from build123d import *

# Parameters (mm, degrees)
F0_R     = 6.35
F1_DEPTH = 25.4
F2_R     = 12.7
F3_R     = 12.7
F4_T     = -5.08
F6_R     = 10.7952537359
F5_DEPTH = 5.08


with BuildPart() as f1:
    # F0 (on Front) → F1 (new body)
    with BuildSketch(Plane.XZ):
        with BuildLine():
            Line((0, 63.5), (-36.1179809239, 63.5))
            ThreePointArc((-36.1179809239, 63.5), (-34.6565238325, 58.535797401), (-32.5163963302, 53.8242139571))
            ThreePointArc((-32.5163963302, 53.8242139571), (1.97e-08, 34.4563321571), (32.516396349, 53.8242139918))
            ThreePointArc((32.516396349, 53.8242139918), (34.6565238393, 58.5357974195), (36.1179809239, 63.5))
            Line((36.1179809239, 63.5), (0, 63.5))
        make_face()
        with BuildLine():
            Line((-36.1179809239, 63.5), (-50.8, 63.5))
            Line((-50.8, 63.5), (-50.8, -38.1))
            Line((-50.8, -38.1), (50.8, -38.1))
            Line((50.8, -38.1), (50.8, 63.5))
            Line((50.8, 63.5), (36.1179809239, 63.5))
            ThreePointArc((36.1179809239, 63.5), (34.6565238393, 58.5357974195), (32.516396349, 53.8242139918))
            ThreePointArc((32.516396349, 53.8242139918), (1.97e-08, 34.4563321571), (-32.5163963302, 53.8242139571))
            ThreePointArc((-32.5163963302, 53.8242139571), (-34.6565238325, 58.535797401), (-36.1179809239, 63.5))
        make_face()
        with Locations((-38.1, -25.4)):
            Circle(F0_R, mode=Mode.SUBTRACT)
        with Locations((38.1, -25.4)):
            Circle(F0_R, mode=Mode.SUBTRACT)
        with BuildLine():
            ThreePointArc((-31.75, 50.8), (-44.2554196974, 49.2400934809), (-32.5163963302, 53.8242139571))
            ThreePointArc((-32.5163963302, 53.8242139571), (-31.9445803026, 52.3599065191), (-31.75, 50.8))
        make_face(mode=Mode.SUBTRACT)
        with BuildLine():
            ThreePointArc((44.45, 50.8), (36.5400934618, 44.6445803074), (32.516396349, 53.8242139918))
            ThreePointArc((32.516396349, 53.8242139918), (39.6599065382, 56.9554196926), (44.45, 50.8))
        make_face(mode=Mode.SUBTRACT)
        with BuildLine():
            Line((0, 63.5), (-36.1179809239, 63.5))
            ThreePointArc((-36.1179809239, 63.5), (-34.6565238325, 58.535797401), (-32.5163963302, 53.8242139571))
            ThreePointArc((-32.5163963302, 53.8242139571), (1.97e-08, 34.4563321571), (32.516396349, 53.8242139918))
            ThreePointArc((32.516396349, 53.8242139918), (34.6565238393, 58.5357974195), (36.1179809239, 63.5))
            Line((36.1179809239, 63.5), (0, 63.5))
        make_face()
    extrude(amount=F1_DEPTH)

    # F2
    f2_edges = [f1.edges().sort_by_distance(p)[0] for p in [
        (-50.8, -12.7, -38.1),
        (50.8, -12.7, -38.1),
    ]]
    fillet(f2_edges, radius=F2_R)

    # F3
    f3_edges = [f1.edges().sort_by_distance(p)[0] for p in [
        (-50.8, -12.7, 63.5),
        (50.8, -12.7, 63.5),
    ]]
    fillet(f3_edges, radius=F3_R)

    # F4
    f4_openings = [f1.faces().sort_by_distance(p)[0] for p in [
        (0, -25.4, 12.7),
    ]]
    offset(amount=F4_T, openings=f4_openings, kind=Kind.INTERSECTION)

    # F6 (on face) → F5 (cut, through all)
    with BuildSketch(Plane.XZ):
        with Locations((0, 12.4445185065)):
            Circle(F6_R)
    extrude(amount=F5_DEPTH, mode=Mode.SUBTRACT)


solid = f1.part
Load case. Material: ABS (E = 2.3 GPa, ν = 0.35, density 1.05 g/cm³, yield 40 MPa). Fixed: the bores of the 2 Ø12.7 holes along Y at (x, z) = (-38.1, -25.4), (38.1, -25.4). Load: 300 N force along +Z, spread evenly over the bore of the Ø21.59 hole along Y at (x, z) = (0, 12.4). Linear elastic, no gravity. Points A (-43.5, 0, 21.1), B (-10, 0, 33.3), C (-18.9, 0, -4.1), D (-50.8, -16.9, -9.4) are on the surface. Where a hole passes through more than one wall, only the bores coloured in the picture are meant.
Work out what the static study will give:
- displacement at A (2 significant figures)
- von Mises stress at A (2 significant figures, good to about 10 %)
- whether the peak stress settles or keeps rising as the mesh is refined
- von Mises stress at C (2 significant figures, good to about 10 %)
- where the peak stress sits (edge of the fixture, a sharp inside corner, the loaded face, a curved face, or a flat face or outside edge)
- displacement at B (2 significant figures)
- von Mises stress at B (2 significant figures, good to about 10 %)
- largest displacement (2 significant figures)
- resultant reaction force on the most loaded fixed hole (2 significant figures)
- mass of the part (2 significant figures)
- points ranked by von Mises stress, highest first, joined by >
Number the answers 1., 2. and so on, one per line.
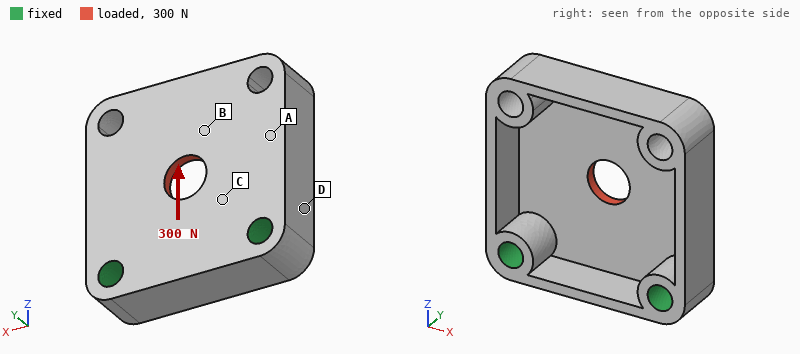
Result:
1. 15 µm
2. 0.30 MPa
3. keeps rising
4. 0.77 MPa
5. edge of the fixture
6. 24 µm
7. 0.55 MPa
8. 37 µm
9. 160 N
10. 110 g
11. C > B > A > D
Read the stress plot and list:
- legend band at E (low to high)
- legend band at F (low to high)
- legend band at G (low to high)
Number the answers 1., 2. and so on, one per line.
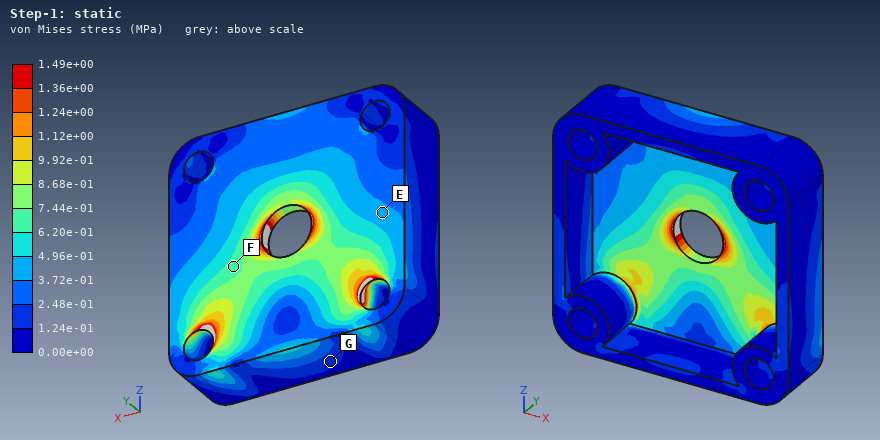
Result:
1. 3.72e-01 to 4.96e-01 MPa
2. 6.20e-01 to 7.44e-01 MPa
3. 1.24e-01 to 2.48e-01 MPa
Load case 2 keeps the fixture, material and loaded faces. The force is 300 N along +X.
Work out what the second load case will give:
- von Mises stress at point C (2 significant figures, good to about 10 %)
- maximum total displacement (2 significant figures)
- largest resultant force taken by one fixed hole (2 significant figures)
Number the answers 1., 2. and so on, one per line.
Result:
1. 0.99 MPa
2. 66 µm
3. 190 N
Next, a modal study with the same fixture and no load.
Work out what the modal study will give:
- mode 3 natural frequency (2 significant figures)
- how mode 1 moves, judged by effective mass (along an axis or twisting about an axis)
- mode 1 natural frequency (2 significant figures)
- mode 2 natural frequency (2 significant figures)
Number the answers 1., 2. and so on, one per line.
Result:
1. 1400 Hz
2. along Y
3. 440 Hz
4. 640 Hz
